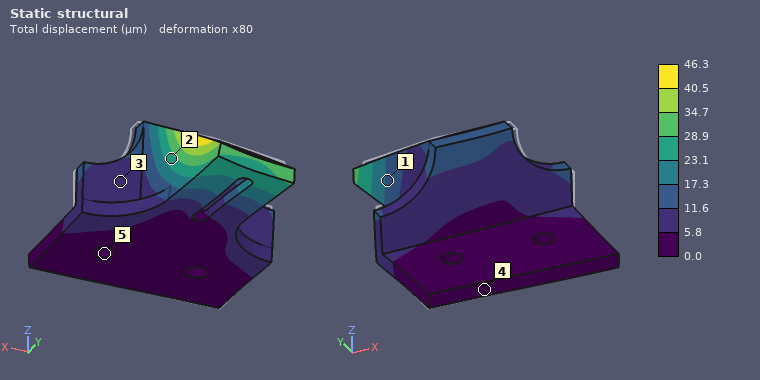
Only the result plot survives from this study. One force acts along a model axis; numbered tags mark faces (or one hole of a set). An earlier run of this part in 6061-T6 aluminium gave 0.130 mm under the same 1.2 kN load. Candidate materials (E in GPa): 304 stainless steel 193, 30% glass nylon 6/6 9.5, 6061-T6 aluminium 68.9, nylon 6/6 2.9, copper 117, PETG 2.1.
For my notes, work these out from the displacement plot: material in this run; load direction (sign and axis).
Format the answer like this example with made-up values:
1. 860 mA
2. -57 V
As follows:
1. 304 stainless steel
2. -X
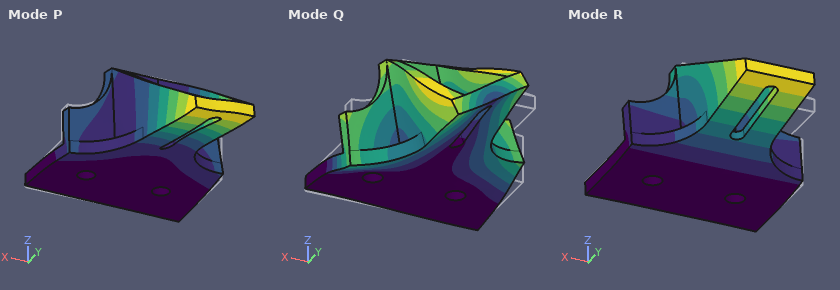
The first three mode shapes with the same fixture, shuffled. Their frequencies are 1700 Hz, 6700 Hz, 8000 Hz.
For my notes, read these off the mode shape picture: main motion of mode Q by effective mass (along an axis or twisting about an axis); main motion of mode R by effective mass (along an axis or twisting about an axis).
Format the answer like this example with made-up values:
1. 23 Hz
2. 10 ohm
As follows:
1. along X
2. along Z
